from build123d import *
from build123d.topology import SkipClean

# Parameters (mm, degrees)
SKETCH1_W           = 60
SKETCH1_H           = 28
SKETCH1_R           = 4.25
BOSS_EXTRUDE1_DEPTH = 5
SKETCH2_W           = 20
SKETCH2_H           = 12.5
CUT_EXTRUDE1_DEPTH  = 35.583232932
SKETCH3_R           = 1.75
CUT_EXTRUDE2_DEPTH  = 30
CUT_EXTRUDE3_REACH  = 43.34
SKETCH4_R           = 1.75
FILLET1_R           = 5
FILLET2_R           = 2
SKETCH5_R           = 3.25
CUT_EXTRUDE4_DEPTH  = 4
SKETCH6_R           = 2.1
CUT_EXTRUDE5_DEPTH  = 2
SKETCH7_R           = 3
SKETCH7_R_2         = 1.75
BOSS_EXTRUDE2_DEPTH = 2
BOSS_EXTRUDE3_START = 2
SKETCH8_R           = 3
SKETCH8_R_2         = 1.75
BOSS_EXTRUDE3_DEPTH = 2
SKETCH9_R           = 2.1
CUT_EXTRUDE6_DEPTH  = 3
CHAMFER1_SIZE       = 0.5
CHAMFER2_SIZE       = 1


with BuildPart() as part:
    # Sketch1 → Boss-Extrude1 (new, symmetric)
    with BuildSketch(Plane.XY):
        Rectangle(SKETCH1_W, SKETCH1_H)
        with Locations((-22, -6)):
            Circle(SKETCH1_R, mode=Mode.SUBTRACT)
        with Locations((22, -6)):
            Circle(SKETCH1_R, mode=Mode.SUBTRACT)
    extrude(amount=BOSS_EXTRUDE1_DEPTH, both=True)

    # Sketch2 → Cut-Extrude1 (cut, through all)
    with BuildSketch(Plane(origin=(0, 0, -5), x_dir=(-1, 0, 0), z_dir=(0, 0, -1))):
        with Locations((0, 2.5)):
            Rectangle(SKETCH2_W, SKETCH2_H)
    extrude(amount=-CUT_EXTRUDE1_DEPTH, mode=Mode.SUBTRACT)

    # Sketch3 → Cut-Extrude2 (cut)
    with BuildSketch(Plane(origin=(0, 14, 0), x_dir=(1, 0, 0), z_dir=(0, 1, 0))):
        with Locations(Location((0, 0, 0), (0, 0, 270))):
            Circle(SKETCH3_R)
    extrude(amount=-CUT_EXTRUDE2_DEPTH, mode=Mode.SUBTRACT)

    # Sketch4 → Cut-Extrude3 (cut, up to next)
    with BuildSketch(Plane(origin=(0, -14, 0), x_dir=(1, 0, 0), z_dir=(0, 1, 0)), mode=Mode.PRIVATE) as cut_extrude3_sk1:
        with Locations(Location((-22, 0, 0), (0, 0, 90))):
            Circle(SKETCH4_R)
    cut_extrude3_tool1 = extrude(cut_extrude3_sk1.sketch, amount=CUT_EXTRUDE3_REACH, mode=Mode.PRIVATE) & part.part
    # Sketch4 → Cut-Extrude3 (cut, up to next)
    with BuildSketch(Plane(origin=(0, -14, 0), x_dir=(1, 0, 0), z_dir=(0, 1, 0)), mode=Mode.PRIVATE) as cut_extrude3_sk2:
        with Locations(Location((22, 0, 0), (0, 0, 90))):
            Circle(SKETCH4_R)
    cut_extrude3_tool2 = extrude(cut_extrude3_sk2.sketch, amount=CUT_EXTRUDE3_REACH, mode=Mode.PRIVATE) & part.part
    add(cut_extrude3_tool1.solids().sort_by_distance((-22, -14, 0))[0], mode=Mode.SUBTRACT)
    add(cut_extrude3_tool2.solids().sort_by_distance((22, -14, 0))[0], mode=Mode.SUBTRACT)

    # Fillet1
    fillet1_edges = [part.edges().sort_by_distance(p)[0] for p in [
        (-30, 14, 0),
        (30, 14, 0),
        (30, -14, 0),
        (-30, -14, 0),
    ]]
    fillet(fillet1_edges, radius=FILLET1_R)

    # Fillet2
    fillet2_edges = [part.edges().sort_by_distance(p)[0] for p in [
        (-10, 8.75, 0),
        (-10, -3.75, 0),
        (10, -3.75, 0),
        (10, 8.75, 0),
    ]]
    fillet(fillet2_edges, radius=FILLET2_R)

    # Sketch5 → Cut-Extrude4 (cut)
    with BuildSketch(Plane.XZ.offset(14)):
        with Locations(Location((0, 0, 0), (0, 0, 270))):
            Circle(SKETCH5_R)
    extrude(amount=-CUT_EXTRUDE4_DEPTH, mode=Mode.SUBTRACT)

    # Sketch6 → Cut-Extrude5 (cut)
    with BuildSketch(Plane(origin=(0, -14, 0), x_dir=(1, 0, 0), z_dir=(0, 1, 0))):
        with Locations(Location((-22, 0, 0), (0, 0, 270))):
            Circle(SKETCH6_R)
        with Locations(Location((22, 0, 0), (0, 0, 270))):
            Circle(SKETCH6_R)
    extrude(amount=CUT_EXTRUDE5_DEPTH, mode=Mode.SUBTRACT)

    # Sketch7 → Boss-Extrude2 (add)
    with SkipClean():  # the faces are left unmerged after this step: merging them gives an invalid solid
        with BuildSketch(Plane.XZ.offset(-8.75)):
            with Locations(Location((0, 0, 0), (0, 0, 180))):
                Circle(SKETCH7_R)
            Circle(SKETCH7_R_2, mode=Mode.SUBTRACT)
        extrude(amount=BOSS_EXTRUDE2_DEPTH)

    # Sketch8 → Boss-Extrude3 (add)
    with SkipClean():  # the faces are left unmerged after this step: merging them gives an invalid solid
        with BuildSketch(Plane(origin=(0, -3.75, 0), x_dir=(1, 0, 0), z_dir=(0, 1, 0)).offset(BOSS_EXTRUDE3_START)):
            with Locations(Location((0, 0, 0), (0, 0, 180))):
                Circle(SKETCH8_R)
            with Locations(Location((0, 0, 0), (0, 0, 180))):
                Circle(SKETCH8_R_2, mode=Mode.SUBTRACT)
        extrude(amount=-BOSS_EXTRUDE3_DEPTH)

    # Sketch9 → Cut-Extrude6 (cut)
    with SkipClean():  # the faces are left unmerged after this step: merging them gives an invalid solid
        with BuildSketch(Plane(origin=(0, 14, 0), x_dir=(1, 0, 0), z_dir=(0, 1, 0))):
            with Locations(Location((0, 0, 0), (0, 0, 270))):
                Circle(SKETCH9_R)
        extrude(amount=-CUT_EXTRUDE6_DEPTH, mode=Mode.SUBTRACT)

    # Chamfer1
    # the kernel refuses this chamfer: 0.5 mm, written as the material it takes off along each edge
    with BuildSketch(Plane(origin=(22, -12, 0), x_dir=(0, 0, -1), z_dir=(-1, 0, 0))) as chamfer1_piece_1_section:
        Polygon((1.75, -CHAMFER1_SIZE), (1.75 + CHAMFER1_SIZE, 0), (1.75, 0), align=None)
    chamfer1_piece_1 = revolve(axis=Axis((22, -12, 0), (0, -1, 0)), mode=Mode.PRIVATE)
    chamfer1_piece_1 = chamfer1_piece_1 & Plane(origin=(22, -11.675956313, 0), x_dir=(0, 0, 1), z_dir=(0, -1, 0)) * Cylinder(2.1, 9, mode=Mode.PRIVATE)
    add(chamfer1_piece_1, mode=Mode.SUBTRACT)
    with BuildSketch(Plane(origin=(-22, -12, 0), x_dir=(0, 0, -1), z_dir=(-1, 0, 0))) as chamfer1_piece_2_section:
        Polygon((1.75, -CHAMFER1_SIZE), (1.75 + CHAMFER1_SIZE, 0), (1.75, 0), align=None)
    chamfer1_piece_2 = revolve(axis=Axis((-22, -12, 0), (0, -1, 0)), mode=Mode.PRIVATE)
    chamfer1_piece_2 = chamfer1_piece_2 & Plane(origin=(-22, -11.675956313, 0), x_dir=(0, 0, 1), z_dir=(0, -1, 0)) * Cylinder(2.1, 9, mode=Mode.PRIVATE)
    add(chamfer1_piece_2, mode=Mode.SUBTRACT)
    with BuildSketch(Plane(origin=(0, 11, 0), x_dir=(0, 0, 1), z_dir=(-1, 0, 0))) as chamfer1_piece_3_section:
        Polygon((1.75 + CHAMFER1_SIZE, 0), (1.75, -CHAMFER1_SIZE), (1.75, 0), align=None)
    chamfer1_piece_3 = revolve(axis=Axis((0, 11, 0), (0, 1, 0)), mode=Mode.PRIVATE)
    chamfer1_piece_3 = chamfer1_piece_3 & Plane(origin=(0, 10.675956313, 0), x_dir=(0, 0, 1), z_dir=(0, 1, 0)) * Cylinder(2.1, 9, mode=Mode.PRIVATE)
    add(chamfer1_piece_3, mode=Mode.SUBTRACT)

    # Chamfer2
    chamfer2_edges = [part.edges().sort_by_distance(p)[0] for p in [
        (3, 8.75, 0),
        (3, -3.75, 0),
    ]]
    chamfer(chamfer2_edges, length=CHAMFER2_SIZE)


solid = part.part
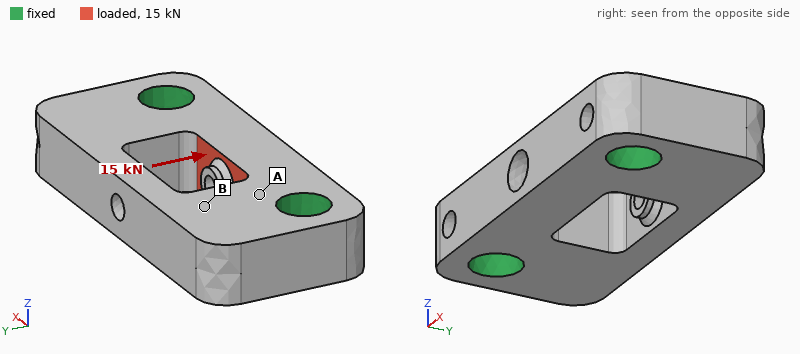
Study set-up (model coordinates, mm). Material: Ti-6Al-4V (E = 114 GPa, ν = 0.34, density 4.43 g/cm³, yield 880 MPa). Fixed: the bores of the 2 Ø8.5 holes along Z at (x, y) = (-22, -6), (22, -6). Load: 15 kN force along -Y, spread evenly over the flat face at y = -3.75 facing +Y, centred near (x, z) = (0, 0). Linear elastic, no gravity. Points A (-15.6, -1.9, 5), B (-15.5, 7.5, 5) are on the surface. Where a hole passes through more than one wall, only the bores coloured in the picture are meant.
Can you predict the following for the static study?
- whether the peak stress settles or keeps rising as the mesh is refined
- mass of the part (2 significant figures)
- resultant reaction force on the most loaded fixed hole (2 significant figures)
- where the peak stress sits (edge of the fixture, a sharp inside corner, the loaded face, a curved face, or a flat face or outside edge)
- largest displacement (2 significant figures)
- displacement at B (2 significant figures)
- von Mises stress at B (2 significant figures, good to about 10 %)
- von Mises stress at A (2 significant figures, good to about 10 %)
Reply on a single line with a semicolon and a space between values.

keeps rising; 56 g; 7.5 kN; a sharp inside corner; 47 µm; 8.2 µm; 39 MPa; 93 MPa
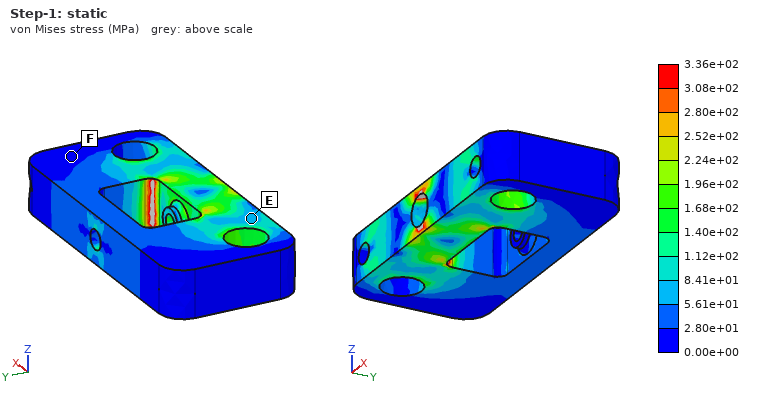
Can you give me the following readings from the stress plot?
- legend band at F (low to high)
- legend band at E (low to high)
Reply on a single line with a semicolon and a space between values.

0.00e+00 to 2.80e+01 MPa; 5.61e+01 to 8.41e+01 MPa
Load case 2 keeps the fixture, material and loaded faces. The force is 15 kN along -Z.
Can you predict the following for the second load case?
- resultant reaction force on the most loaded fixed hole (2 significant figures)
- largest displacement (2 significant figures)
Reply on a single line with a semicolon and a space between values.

7.5 kN; 89 µm
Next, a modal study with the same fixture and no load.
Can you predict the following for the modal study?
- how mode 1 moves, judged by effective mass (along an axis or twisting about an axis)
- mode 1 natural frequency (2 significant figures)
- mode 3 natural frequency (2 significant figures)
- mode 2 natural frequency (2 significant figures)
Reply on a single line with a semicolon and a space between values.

along Z; 16 kHz; 24 kHz; 23 kHz
